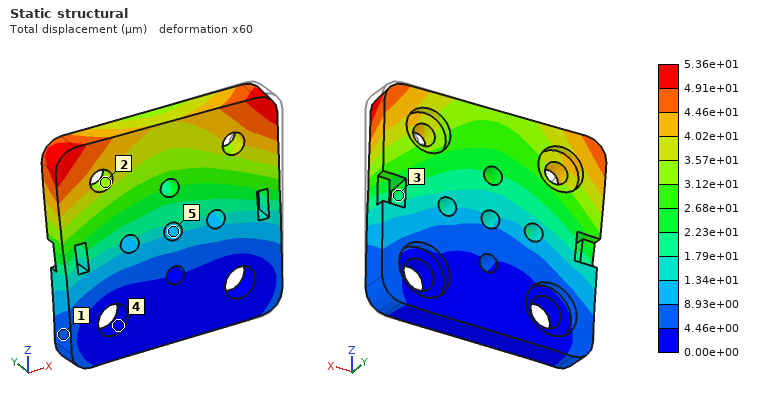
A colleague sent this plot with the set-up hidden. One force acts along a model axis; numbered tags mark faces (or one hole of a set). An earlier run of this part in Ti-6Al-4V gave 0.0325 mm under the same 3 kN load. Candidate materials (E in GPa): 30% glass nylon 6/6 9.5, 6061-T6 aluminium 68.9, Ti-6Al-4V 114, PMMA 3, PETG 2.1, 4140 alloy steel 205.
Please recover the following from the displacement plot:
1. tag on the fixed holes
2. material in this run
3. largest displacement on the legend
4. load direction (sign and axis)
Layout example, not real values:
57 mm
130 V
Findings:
4
6061-T6 aluminium
5.36e+01 µm
-X
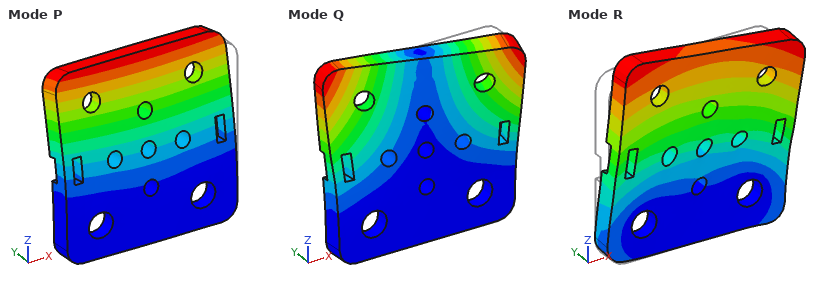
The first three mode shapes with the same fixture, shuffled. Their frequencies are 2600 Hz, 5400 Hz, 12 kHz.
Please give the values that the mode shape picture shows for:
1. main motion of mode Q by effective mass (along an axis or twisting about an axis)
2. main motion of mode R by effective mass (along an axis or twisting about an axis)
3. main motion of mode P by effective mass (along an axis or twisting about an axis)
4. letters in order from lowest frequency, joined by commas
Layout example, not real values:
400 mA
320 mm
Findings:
twisting about Z
along X
along Y
P, Q, R
